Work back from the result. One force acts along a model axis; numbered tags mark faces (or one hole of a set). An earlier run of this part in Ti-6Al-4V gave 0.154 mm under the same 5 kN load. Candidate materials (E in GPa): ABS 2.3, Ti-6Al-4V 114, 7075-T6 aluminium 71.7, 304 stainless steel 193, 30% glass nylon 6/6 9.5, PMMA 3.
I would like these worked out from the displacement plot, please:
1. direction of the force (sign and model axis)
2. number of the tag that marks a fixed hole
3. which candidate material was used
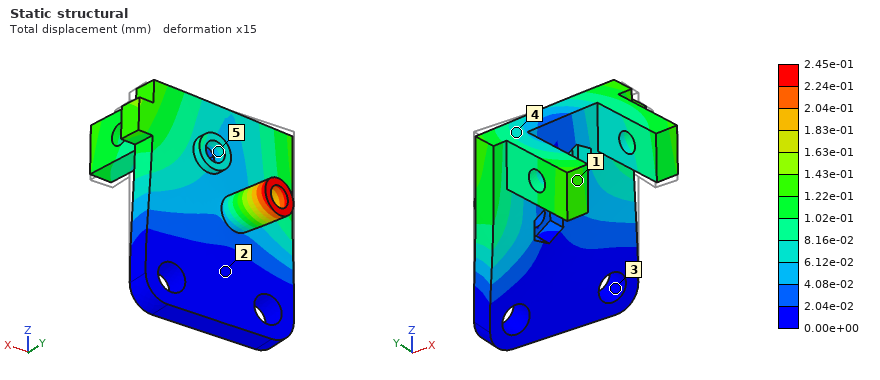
-X
3
7075-T6 aluminium
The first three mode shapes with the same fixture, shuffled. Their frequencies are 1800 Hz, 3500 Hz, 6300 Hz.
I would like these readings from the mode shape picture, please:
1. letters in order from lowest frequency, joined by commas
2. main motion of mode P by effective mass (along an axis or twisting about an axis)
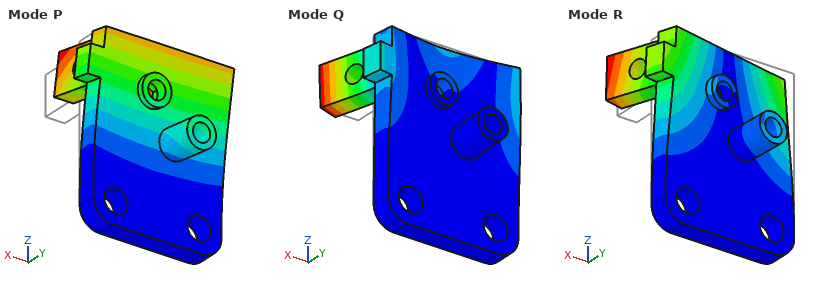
P, R, Q
along Y
